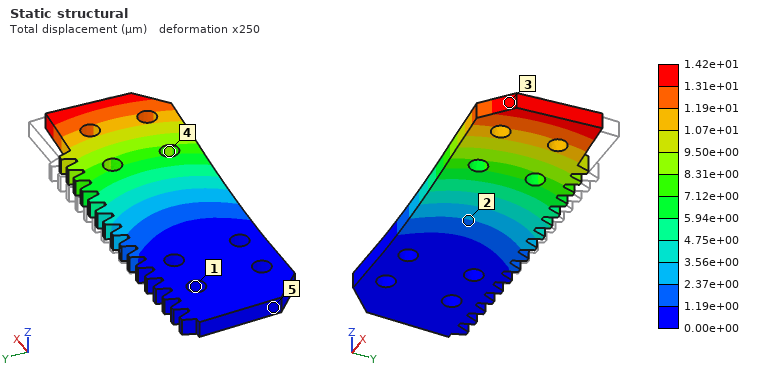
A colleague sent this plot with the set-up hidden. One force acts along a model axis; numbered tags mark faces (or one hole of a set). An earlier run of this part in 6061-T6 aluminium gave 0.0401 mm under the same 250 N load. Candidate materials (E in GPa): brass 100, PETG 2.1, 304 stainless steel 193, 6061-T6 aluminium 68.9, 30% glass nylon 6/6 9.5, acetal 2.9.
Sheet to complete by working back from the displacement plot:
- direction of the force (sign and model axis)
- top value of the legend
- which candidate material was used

-Y
1.42e+01 µm
304 stainless steel
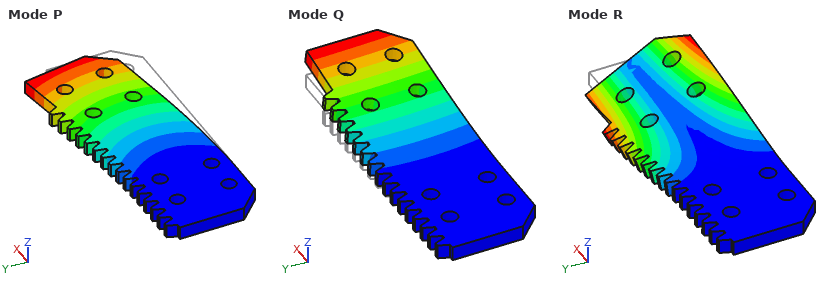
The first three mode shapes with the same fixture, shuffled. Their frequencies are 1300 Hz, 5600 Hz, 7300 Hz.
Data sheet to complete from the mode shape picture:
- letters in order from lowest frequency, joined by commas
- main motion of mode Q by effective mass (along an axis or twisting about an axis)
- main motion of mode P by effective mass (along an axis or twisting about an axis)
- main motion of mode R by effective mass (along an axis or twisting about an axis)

Q, R, P
along Z
along Y
twisting about X
